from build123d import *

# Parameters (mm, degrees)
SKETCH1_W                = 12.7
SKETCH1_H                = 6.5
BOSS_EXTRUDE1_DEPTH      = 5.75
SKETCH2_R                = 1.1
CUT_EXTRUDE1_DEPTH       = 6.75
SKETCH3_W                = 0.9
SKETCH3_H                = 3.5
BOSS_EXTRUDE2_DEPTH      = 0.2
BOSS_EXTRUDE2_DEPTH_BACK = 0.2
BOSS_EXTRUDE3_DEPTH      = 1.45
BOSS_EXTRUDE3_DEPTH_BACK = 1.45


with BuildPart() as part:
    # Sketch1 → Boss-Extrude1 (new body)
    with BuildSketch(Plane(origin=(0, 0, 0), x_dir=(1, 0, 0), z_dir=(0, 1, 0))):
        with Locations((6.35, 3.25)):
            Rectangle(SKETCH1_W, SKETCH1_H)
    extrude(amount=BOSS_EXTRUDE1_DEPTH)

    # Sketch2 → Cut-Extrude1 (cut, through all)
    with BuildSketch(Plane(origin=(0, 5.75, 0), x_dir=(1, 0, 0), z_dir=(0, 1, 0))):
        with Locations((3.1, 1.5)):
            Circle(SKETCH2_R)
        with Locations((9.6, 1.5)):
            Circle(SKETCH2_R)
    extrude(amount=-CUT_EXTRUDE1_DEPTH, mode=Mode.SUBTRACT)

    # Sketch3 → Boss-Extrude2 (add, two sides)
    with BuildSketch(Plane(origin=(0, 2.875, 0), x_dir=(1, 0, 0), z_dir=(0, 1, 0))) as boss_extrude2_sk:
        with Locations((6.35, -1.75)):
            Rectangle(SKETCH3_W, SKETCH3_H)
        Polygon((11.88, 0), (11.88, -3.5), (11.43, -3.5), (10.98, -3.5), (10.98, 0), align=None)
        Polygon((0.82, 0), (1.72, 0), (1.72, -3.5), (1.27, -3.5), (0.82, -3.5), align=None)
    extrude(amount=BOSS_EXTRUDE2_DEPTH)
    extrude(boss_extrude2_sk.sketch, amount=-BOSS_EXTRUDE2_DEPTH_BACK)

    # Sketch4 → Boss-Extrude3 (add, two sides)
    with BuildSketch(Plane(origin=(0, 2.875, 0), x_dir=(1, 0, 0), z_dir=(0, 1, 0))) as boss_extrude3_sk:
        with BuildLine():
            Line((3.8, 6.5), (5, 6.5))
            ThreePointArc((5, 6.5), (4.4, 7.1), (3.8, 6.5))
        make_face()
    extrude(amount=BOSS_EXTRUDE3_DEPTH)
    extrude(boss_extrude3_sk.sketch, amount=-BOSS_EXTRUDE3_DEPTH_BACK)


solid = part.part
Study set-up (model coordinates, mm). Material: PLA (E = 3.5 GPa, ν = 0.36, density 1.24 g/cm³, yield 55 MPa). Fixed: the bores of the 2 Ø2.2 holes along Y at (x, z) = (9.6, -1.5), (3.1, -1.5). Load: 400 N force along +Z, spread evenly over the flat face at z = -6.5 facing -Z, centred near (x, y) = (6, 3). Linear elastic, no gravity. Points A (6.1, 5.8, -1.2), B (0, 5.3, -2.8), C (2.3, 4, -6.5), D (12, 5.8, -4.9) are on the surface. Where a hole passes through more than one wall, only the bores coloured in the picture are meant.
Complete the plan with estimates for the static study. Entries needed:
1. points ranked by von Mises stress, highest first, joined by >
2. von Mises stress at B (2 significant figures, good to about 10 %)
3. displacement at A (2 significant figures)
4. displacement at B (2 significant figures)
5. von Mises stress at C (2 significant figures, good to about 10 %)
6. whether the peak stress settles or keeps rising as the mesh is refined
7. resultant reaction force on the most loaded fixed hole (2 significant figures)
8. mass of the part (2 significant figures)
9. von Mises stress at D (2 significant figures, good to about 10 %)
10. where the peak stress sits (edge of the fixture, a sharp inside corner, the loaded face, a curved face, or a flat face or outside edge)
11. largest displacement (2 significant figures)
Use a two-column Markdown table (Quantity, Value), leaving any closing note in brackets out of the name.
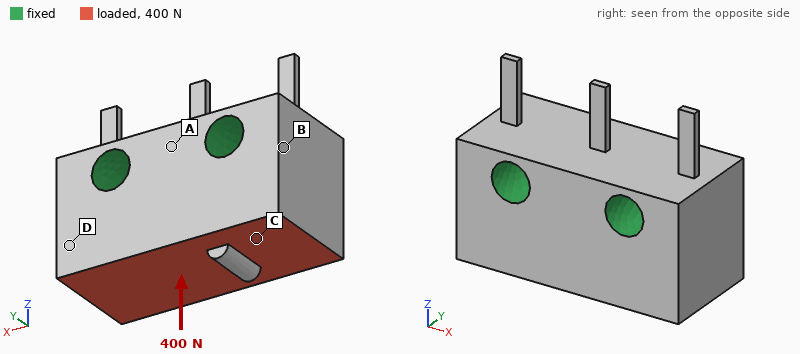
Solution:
| Quantity | Value |
|---|---|
| points ranked by von Mises stress, highest first, joined by > | C > D > B > A |
| von Mises stress at B | 2.5 MPa |
| displacement at A | 3.2 µm |
| displacement at B | 6.3 µm |
| von Mises stress at C | 6.6 MPa |
| whether the peak stress settles or keeps rising as the mesh is refined | keeps rising |
| resultant reaction force on the most loaded fixed hole | 210 N |
| mass of the part | 0.54 g |
| von Mises stress at D | 5.1 MPa |
| where the peak stress sits | edge of the fixture |
| largest displacement | 12 µm |
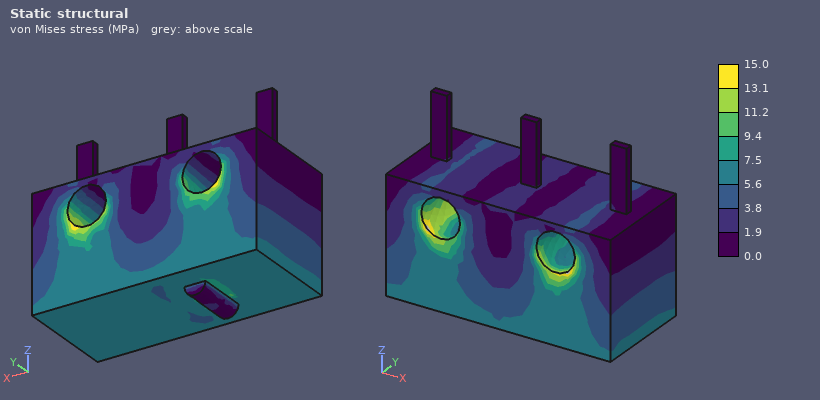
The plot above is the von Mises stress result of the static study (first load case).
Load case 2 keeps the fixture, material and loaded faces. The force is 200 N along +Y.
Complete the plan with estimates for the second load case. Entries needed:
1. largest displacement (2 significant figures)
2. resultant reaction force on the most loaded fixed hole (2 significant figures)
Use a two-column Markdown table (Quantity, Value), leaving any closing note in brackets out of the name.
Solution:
| Quantity | Value |
|---|---|
| largest displacement | 27 µm |
| resultant reaction force on the most loaded fixed hole | 100 N |
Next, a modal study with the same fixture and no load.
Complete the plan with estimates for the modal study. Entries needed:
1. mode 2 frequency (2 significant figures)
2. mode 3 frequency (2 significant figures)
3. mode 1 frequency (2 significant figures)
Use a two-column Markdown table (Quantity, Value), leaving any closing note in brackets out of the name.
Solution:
| Quantity | Value |
|---|---|
| mode 2 frequency | 8500 Hz |
| mode 3 frequency | 8500 Hz |
| mode 1 frequency | 8500 Hz |
